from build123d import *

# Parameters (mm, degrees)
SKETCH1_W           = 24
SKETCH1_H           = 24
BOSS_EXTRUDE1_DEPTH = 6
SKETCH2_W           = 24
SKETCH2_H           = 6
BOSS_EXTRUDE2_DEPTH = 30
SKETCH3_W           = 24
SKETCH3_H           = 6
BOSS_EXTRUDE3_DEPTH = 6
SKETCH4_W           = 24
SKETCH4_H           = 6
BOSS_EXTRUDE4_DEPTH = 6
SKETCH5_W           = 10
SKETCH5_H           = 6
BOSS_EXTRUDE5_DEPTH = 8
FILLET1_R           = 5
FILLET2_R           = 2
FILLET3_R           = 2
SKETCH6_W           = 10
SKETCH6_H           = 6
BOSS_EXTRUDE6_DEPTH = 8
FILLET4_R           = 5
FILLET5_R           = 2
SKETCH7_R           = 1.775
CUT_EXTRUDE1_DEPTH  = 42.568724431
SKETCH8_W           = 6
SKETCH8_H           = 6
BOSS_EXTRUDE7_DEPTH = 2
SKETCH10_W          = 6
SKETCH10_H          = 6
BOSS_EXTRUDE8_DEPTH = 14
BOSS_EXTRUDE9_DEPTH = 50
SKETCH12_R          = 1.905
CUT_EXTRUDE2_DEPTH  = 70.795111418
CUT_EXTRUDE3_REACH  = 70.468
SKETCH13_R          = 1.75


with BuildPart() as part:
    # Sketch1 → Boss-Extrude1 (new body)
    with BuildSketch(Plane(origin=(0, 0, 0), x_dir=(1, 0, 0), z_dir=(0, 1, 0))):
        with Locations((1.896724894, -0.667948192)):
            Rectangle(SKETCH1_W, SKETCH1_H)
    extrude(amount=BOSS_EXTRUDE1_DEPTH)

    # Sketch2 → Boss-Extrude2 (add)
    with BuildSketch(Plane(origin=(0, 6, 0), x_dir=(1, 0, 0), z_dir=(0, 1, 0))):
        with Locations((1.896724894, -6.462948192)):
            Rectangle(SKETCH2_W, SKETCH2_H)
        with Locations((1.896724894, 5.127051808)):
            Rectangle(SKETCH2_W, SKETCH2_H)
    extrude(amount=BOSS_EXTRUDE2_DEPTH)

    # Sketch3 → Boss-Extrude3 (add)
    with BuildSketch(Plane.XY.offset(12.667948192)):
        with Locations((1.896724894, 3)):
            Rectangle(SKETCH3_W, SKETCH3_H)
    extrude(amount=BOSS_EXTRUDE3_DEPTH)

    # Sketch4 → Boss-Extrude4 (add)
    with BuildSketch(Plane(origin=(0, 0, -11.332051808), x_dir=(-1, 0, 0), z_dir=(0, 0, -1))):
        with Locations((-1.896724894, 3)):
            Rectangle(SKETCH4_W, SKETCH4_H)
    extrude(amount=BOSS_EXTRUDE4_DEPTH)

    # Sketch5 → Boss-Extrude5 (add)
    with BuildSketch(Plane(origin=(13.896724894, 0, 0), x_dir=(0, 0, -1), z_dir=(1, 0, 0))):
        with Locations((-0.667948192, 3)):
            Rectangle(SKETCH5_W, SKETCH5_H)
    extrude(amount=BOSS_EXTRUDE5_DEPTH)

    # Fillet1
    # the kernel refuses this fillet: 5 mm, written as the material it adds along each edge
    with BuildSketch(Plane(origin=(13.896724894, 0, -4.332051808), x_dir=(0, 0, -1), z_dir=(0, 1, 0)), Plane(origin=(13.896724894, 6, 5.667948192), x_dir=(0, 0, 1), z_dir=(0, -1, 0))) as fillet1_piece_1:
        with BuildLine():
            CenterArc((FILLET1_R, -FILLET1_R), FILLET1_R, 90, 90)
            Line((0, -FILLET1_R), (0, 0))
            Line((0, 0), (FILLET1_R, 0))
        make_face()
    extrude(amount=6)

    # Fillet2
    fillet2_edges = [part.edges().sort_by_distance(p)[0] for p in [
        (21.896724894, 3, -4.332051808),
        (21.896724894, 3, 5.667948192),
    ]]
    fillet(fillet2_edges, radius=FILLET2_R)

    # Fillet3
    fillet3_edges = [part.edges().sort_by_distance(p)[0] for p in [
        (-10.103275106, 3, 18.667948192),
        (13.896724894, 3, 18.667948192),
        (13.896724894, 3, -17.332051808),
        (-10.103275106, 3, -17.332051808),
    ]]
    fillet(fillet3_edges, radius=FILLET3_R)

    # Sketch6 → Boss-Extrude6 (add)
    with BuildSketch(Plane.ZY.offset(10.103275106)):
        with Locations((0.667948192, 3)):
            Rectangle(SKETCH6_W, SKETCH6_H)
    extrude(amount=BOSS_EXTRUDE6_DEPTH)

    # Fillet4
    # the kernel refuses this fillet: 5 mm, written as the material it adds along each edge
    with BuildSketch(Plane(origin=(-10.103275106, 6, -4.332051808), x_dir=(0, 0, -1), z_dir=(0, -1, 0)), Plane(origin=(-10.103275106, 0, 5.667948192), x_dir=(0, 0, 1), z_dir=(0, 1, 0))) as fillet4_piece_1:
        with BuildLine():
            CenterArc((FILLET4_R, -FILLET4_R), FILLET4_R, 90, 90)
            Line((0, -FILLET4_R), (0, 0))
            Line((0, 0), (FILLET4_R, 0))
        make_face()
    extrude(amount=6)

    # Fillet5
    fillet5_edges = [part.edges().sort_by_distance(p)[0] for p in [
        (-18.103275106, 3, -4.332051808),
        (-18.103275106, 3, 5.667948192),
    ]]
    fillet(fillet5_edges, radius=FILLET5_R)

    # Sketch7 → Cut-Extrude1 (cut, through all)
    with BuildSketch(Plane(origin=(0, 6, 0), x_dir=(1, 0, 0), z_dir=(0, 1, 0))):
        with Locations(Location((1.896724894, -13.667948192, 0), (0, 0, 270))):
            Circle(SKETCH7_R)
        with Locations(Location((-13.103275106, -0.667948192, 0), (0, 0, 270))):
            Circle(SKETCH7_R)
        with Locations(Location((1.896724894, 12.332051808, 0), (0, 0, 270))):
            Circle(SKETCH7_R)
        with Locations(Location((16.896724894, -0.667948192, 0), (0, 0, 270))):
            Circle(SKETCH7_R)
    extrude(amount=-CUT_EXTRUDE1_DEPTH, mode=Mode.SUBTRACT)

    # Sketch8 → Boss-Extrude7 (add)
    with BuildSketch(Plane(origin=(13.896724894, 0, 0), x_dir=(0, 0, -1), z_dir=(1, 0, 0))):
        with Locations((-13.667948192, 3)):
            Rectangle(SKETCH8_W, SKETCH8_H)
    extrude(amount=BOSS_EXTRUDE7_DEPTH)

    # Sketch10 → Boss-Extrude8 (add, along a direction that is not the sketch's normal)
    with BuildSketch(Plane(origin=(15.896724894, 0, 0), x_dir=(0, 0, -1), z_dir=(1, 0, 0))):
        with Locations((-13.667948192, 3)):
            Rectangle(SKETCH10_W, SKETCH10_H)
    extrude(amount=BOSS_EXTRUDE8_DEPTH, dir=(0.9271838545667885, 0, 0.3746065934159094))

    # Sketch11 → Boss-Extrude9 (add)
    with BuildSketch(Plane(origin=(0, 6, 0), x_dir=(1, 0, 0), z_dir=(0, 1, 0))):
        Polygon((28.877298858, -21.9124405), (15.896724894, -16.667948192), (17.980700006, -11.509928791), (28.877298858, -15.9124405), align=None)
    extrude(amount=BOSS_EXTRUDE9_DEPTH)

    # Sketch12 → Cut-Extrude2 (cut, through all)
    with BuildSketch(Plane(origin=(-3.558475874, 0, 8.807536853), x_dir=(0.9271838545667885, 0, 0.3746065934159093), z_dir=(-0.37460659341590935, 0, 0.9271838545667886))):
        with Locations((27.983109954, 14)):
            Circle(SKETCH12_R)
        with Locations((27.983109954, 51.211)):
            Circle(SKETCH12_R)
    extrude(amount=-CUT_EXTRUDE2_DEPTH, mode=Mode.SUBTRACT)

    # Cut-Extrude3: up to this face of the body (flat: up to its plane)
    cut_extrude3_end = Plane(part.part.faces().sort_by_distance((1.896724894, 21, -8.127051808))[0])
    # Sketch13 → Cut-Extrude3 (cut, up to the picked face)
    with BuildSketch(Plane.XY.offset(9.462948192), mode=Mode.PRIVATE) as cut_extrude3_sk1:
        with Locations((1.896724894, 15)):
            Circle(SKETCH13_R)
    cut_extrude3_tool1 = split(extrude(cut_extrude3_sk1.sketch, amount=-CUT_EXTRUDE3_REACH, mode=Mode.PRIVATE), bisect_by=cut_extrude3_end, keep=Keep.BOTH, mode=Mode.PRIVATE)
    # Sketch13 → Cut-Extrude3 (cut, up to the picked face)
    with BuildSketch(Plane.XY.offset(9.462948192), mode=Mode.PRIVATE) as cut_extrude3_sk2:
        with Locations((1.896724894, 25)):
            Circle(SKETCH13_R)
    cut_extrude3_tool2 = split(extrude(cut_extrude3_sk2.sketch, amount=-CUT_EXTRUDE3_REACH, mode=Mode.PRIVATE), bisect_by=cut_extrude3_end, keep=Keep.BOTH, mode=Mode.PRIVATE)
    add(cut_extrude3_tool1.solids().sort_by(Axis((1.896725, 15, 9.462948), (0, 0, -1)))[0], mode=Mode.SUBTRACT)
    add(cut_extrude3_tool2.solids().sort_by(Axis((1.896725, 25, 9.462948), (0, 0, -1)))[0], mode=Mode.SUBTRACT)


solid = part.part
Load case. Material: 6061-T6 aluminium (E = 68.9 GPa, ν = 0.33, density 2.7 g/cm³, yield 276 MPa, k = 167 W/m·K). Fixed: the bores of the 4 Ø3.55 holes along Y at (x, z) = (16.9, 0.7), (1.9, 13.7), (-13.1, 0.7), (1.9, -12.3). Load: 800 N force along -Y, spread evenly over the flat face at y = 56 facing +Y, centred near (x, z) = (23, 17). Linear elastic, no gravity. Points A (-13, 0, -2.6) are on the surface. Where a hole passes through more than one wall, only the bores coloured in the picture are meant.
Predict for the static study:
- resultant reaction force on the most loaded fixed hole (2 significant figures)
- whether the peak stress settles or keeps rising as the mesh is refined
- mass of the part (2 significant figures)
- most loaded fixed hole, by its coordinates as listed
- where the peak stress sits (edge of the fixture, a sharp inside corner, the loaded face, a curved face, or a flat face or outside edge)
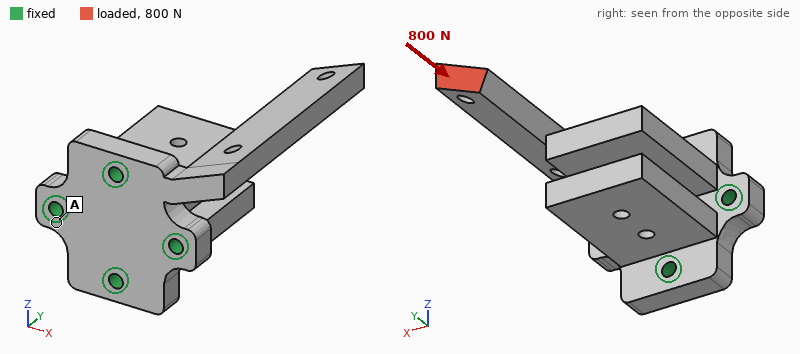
690 N
keeps rising
50 g
(1.9, 13.7)
a sharp inside corner
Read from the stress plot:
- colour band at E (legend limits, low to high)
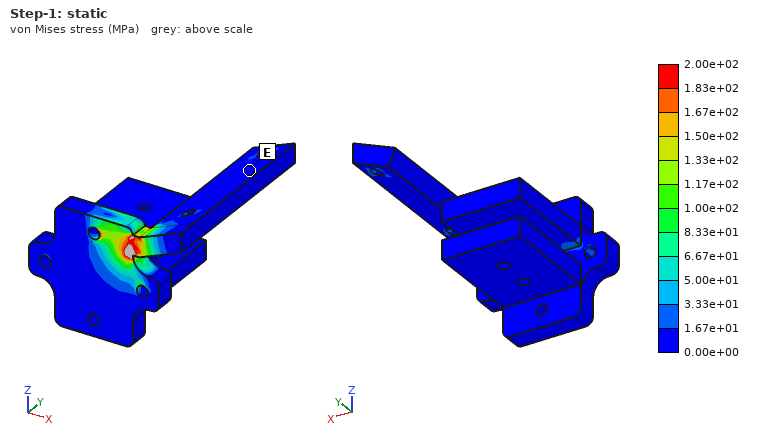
0.00e+00 to 1.67e+01 MPa
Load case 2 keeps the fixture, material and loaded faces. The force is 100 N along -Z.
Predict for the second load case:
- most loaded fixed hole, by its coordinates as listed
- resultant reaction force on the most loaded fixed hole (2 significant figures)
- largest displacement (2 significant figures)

(1.9, 13.7)
300 N
0.87 mm
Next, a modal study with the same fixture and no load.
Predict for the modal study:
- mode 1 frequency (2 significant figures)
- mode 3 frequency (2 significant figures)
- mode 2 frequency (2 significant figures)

1000 Hz
4500 Hz
1200 Hz
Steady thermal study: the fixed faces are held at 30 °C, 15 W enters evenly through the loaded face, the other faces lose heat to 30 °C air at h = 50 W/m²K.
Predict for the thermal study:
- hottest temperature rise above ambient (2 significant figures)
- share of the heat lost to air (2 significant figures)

77 K
34 %
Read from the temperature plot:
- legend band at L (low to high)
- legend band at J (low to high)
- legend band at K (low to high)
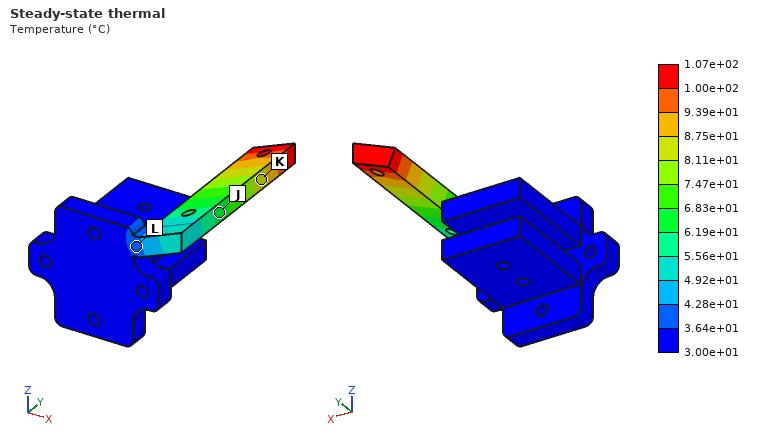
3.64e+01 to 4.28e+01 °C
6.19e+01 to 6.83e+01 °C
8.11e+01 to 8.75e+01 °C
